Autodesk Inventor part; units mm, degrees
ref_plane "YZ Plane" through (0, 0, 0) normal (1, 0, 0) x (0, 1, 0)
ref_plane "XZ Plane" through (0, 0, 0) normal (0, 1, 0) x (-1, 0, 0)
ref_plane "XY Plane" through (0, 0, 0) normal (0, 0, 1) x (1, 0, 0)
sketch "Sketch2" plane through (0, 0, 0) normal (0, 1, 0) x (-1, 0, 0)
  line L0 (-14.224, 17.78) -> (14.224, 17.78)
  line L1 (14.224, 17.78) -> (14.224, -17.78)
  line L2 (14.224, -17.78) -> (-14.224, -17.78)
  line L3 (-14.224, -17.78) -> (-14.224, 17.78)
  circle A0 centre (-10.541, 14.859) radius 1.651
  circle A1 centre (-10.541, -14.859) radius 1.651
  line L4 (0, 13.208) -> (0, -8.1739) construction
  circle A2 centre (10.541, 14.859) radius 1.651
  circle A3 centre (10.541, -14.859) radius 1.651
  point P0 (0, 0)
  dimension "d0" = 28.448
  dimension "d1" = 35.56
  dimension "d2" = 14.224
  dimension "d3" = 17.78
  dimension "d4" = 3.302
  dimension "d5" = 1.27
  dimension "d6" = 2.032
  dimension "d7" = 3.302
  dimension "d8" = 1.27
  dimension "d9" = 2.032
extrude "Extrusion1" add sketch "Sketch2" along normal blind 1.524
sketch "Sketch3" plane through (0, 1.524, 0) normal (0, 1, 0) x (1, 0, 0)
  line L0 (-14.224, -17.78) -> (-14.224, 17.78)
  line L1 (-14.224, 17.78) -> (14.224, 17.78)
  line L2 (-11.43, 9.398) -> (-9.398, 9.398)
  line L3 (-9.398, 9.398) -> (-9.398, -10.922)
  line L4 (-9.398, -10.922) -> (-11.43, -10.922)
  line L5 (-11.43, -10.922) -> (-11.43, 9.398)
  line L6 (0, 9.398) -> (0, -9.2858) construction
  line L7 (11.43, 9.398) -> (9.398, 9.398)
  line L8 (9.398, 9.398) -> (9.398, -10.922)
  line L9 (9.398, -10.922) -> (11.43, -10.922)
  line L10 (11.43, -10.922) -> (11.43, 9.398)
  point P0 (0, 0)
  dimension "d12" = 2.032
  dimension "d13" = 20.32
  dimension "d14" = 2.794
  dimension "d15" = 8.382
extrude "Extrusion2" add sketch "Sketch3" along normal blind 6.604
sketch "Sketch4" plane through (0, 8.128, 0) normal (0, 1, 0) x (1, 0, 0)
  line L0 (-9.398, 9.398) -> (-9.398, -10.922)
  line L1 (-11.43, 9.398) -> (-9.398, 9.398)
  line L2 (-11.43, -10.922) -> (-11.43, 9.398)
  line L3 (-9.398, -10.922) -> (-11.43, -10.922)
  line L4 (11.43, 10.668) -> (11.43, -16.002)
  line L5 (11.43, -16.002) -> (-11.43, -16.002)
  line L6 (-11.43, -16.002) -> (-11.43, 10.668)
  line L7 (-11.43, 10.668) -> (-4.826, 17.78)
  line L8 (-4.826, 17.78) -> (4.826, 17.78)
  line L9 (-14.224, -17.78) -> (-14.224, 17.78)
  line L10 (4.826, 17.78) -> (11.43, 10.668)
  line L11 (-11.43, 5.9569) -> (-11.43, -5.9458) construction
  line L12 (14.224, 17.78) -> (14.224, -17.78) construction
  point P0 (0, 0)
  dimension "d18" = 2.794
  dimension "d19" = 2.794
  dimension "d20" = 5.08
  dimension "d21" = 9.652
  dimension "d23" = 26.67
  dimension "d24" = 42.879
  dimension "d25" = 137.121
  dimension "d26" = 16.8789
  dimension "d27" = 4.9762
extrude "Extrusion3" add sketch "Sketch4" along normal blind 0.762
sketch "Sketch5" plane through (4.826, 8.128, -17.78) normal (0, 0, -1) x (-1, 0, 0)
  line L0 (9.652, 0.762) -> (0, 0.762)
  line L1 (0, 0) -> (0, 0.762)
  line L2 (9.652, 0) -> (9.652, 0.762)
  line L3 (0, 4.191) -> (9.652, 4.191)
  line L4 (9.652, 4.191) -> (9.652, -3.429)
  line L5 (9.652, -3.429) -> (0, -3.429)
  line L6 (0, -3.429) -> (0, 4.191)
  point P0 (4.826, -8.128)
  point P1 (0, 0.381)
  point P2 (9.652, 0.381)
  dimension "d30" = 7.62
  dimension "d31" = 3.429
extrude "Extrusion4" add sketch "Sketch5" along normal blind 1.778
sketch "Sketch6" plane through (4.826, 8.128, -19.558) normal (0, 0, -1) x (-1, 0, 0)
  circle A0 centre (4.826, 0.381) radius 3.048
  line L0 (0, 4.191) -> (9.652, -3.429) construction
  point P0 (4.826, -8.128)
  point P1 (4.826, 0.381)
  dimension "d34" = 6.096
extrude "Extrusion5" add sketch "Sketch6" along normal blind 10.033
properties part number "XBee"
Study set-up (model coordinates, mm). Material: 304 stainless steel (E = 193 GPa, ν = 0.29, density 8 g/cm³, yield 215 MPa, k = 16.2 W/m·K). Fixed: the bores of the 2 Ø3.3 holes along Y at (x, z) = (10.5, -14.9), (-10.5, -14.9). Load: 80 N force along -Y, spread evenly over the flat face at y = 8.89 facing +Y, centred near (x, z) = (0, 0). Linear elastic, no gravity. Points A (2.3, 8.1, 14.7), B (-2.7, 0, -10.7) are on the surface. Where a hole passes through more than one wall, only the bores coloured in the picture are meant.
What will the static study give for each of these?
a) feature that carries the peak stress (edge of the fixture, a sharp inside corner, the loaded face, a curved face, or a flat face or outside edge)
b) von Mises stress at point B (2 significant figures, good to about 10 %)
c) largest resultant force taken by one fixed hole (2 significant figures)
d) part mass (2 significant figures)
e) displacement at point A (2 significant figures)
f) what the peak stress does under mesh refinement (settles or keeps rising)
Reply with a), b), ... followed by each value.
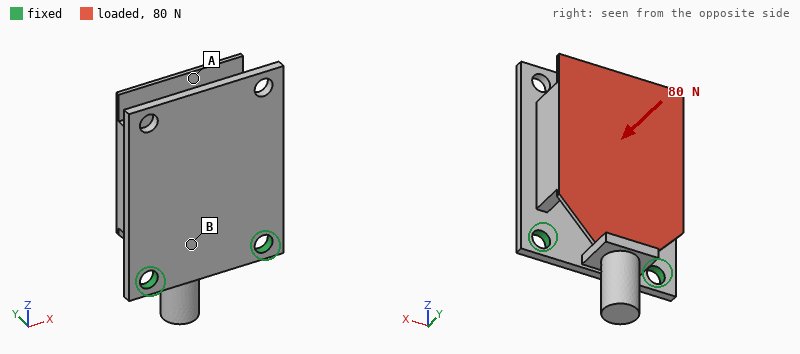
a) edge of the fixture
b) 44 MPa
c) 40 N
d) 24 g
e) 0.12 mm
f) keeps rising
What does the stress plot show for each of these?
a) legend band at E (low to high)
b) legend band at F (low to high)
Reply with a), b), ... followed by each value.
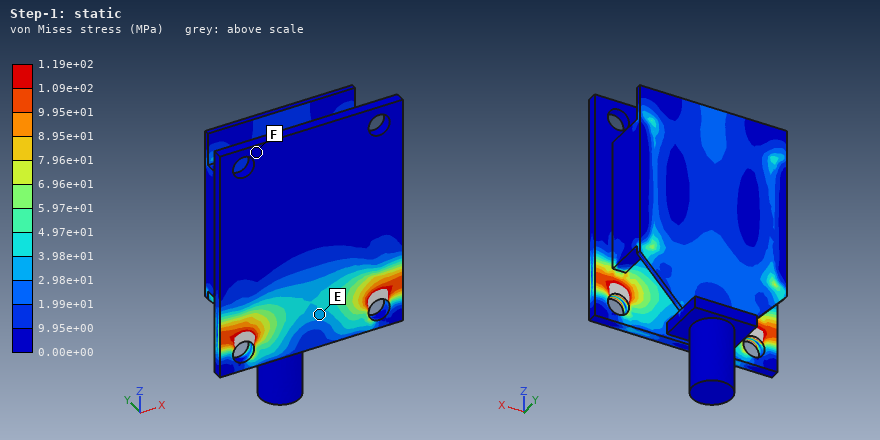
a) 2.98e+01 to 3.98e+01 MPa
b) 0.00e+00 to 9.95e+00 MPa
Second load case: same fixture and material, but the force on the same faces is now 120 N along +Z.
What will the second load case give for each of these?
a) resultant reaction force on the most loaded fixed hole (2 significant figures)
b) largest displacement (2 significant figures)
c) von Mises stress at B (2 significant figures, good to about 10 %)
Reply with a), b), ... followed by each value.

a) 60 N
b) 0.13 mm
c) 50 MPa
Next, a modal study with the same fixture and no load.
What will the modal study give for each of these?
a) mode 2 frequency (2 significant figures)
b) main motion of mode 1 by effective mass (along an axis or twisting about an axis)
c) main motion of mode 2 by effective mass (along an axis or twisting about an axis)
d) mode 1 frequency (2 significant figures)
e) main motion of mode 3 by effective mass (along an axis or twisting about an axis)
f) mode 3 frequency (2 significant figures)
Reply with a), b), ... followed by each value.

a) 1100 Hz
b) twisting about X
c) along Y
d) 760 Hz
e) along X
f) 3300 Hz
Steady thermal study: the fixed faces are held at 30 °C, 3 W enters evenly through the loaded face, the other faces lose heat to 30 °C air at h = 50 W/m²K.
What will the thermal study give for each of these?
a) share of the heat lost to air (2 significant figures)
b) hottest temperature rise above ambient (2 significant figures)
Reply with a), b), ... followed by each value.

a) 81 %
b) 33 K
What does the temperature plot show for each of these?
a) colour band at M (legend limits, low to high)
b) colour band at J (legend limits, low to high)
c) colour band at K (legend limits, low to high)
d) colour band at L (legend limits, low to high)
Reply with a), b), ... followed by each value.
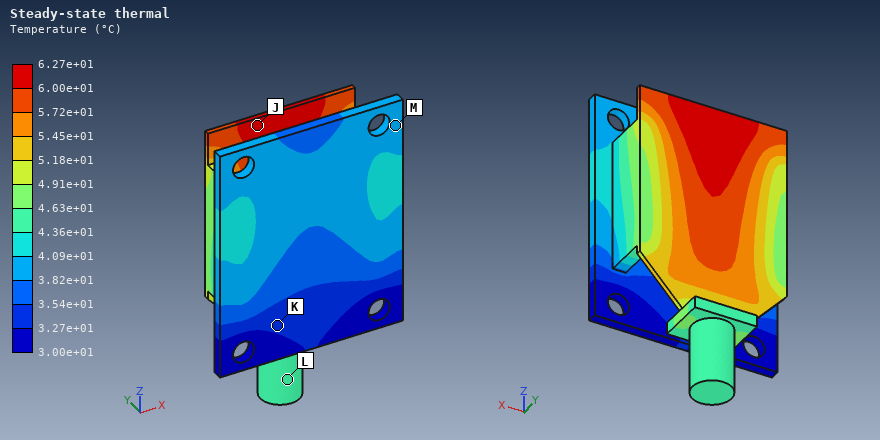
a) 3.82e+01 to 4.09e+01 °C
b) 6.00e+01 to 6.27e+01 °C
c) 3.27e+01 to 3.54e+01 °C
d) 4.36e+01 to 4.63e+01 °C
